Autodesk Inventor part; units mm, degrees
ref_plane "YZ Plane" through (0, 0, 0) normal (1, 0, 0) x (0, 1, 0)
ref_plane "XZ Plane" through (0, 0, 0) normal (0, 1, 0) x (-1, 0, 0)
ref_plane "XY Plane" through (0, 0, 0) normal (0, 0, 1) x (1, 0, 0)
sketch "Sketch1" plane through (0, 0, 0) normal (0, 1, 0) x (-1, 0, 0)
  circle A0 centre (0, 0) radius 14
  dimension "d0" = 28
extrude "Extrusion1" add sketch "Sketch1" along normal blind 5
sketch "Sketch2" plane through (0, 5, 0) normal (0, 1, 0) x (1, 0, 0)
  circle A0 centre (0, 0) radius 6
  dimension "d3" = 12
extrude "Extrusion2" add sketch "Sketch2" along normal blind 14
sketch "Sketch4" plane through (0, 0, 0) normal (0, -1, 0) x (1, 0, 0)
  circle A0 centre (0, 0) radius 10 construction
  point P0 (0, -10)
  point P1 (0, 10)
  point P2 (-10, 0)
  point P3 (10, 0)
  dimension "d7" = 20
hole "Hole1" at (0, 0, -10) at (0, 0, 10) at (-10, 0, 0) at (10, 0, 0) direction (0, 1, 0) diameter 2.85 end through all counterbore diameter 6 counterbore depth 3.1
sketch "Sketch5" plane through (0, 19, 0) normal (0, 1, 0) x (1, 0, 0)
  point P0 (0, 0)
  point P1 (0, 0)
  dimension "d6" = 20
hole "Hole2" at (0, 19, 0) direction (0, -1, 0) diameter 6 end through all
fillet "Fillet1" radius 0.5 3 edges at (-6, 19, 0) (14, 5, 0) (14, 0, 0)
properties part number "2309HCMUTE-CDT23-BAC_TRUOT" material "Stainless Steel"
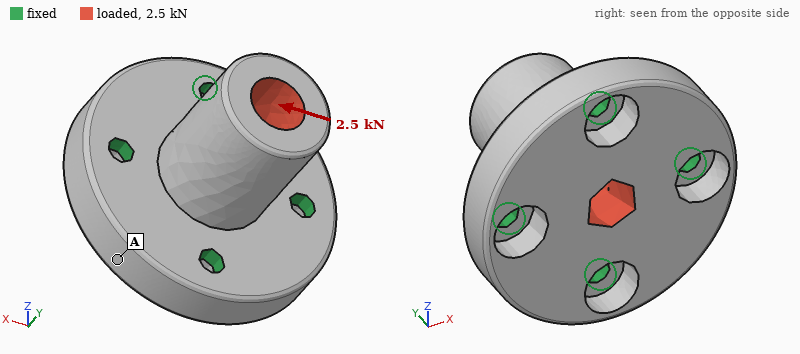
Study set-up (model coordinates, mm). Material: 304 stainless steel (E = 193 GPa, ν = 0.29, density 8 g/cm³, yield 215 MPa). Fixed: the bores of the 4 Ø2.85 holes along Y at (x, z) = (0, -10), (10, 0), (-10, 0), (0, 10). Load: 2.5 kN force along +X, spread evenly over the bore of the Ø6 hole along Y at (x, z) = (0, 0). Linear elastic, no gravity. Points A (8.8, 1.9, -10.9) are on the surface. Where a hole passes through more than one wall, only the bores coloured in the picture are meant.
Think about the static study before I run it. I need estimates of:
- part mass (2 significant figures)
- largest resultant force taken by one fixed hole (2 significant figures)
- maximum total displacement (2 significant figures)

30 g
960 N
15 µm
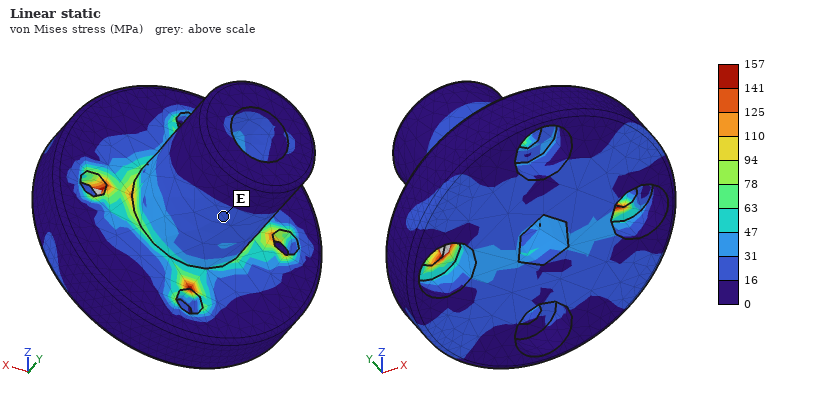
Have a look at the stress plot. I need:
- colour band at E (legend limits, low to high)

16 to 31 MPa
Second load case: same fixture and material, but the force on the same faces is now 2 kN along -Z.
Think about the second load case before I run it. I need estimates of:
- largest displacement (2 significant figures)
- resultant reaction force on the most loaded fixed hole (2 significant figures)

12 µm
770 N
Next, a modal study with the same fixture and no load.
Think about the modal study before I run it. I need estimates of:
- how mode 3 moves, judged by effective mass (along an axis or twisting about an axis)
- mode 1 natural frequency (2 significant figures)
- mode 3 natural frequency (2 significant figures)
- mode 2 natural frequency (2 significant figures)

along Y
21 kHz
34 kHz
21 kHz
